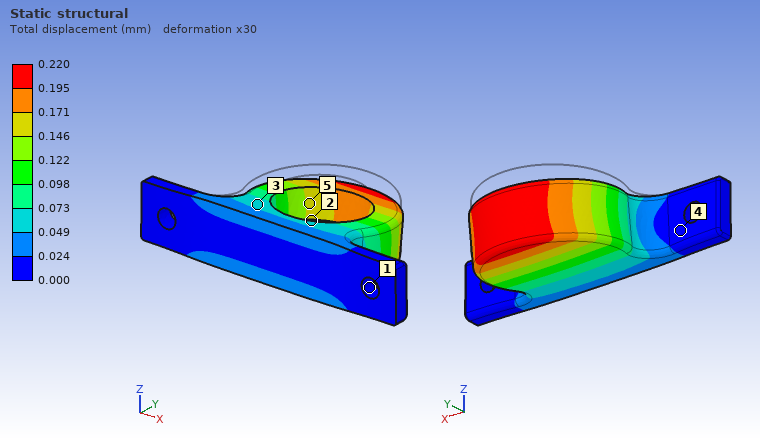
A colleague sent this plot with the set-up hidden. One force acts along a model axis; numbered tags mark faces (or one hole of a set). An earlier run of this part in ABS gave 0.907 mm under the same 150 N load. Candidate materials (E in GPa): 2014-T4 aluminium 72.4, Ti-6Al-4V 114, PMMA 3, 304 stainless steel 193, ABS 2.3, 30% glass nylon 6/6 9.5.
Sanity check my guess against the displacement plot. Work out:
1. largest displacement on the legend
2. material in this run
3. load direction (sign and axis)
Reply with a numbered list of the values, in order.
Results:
1. 0.220 mm
2. 30% glass nylon 6/6
3. -Z
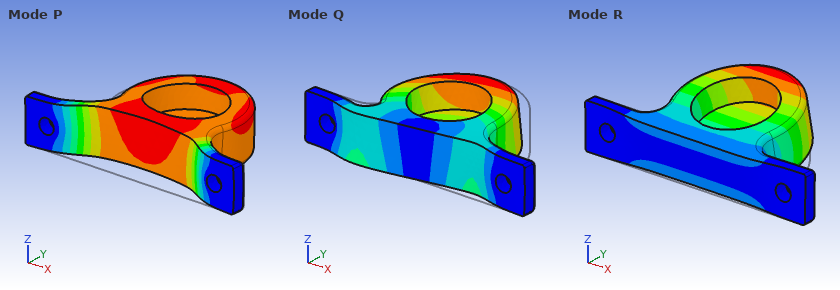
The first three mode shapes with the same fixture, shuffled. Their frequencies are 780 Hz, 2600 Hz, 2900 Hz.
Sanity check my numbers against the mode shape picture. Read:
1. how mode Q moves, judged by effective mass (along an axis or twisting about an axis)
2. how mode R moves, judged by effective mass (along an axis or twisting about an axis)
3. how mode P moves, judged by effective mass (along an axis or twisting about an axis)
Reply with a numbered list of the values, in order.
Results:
1. along X
2. along Z
3. along Y
